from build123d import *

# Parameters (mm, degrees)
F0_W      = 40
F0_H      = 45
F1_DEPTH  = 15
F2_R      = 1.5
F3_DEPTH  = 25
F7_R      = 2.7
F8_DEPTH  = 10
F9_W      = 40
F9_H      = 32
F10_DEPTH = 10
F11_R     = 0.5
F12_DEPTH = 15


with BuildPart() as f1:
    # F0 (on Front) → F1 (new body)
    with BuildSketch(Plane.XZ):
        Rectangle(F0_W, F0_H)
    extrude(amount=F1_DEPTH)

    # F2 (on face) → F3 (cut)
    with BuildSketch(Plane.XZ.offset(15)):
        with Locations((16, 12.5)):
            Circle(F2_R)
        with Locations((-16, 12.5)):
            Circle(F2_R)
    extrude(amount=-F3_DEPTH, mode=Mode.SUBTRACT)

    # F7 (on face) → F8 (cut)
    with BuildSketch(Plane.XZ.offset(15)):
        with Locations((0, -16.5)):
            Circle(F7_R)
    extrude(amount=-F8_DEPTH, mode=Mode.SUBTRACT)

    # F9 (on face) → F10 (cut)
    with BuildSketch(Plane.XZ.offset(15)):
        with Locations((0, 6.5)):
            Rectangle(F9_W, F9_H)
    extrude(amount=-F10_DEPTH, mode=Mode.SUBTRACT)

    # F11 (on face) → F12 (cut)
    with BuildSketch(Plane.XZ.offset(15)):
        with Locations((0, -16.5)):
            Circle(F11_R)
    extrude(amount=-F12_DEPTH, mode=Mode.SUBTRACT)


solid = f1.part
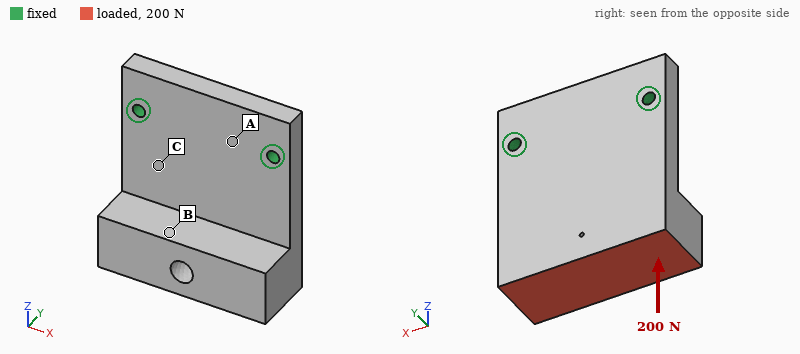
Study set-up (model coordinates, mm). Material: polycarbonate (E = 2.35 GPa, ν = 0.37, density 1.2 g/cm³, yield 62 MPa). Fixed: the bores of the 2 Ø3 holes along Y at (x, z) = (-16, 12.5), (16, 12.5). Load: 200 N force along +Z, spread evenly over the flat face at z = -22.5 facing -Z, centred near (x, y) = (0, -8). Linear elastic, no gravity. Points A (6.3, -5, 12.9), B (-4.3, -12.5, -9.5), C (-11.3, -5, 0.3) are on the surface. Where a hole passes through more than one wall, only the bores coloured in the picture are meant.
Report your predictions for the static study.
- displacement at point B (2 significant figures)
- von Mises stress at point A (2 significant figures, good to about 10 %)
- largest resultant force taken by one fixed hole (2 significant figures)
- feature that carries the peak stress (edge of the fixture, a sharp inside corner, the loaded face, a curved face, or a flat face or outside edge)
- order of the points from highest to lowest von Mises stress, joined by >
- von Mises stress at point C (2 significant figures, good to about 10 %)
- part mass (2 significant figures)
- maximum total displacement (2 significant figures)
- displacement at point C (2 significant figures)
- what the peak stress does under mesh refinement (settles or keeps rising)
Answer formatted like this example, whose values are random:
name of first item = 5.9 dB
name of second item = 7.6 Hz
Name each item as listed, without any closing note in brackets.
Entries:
displacement at point B = 0.41 mm
von Mises stress at point A = 3.0 MPa
largest resultant force taken by one fixed hole = 100 N
feature that carries the peak stress = edge of the fixture
order of the points from highest to lowest von Mises stress, joined by > = C > A > B
von Mises stress at point C = 6.6 MPa
part mass = 17 g
maximum total displacement = 0.73 mm
displacement at point C = 0.12 mm
what the peak stress does under mesh refinement = keeps rising
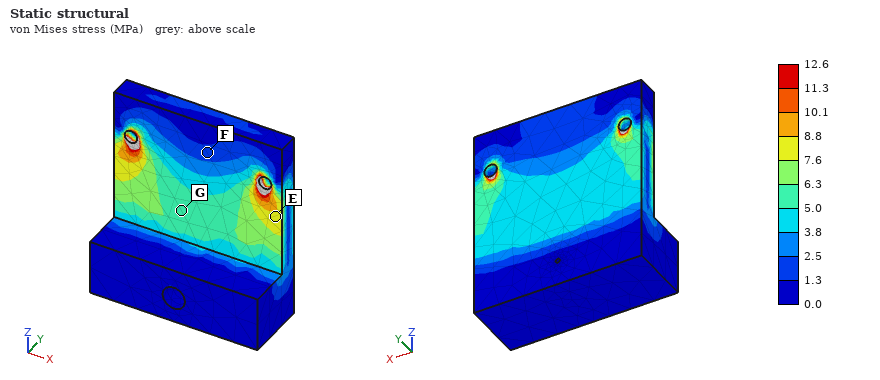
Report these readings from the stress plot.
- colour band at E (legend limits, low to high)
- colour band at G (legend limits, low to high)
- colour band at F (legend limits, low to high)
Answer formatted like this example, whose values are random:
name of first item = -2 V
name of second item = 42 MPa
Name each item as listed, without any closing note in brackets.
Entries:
colour band at E = 7.6 to 8.8 MPa
colour band at G = 5.0 to 6.3 MPa
colour band at F = 1.3 to 2.5 MPa
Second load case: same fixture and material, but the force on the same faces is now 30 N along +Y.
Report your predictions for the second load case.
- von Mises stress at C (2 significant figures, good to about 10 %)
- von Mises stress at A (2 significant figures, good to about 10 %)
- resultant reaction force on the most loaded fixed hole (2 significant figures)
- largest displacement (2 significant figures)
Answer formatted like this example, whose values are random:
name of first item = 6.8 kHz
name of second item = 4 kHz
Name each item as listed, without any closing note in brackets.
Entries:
von Mises stress at C = 3.9 MPa
von Mises stress at A = 2.5 MPa
resultant reaction force on the most loaded fixed hole = 15 N
largest displacement = 0.57 mm
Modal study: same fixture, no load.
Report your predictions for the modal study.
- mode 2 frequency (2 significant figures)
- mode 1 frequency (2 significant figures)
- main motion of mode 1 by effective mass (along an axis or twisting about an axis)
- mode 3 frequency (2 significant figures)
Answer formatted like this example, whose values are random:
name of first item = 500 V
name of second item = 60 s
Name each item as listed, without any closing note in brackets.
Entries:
mode 2 frequency = 1400 Hz
mode 1 frequency = 480 Hz
main motion of mode 1 by effective mass = along Y
mode 3 frequency = 2800 Hz
